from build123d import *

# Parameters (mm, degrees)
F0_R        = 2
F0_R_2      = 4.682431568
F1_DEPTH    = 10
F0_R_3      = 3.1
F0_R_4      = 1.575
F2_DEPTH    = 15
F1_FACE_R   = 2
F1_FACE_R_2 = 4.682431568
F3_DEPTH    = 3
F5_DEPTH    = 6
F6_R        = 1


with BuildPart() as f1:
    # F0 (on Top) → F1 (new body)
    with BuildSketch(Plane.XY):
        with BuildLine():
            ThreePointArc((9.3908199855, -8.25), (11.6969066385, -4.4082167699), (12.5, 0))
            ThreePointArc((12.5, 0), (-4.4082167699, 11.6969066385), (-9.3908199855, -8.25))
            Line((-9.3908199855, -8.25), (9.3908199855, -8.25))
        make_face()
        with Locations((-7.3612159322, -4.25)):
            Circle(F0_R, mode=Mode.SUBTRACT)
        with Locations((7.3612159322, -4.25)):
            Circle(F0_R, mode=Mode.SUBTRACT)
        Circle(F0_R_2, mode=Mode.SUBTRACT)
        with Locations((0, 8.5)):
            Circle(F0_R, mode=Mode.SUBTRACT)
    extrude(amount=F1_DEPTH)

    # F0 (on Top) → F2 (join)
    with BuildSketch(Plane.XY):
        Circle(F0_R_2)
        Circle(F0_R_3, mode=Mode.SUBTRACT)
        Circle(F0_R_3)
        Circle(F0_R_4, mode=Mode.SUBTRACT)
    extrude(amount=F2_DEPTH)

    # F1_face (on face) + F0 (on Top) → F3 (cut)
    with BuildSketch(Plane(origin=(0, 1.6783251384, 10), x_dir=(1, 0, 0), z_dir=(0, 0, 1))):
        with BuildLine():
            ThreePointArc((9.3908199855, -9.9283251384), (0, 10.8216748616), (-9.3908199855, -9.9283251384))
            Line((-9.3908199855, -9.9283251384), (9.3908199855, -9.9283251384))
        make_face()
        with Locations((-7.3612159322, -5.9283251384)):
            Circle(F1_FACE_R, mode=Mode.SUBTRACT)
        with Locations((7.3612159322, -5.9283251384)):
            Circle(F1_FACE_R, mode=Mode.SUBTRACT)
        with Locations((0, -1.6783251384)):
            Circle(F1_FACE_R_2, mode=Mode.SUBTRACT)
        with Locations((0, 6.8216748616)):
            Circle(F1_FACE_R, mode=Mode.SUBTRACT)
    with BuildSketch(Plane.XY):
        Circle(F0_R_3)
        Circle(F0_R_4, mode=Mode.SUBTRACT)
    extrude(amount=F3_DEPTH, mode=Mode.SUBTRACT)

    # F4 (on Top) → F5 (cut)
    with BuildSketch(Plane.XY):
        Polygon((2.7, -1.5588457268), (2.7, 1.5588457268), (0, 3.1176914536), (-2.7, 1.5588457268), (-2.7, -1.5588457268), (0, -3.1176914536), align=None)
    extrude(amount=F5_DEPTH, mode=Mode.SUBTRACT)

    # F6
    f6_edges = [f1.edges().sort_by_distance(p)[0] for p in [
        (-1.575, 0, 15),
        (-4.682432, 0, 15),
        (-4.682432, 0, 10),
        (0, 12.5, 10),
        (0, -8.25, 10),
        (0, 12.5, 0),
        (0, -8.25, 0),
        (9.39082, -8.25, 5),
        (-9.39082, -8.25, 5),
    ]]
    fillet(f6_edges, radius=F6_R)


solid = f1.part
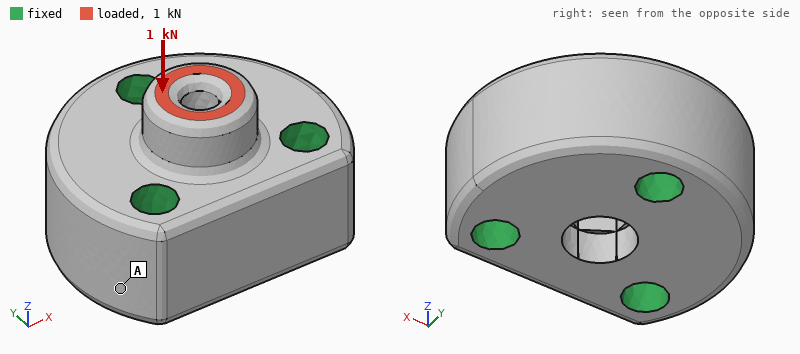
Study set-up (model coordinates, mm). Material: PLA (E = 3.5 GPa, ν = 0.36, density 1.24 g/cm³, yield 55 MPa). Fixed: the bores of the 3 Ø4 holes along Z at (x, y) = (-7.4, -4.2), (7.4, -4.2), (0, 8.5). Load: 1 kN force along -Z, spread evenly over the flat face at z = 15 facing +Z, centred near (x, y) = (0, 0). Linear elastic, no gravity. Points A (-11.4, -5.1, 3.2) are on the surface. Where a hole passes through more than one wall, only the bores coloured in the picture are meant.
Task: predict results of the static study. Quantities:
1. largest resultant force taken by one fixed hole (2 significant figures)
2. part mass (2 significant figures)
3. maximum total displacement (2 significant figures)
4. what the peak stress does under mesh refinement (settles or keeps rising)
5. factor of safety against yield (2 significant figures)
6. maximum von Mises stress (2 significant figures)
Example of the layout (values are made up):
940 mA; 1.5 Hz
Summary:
360 N; 5.0 g; 48 µm; settles; 1.6; 35 MPa
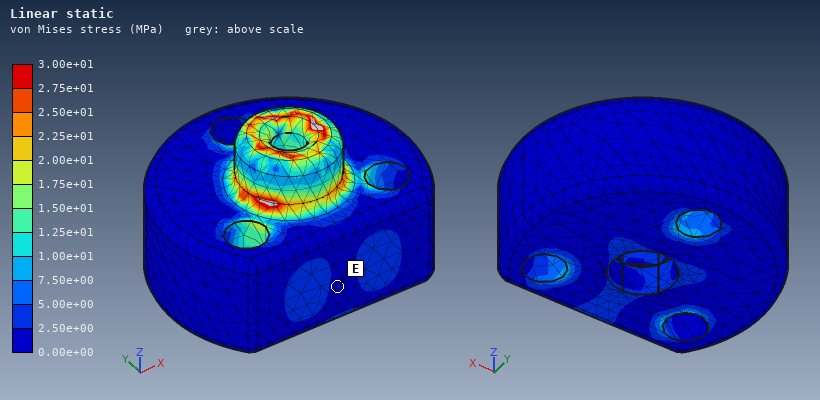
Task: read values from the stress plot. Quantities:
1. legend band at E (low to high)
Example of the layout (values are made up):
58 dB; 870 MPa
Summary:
0.00e+00 to 2.50e+00 MPa
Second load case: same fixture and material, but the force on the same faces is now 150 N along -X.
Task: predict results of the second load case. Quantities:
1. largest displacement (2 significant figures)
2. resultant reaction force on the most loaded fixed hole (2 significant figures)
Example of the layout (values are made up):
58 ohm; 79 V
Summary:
30 µm; 93 N
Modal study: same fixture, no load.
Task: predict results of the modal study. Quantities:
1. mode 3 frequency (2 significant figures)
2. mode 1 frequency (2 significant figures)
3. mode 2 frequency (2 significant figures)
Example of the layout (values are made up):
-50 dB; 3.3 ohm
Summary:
29 kHz; 24 kHz; 25 kHz
